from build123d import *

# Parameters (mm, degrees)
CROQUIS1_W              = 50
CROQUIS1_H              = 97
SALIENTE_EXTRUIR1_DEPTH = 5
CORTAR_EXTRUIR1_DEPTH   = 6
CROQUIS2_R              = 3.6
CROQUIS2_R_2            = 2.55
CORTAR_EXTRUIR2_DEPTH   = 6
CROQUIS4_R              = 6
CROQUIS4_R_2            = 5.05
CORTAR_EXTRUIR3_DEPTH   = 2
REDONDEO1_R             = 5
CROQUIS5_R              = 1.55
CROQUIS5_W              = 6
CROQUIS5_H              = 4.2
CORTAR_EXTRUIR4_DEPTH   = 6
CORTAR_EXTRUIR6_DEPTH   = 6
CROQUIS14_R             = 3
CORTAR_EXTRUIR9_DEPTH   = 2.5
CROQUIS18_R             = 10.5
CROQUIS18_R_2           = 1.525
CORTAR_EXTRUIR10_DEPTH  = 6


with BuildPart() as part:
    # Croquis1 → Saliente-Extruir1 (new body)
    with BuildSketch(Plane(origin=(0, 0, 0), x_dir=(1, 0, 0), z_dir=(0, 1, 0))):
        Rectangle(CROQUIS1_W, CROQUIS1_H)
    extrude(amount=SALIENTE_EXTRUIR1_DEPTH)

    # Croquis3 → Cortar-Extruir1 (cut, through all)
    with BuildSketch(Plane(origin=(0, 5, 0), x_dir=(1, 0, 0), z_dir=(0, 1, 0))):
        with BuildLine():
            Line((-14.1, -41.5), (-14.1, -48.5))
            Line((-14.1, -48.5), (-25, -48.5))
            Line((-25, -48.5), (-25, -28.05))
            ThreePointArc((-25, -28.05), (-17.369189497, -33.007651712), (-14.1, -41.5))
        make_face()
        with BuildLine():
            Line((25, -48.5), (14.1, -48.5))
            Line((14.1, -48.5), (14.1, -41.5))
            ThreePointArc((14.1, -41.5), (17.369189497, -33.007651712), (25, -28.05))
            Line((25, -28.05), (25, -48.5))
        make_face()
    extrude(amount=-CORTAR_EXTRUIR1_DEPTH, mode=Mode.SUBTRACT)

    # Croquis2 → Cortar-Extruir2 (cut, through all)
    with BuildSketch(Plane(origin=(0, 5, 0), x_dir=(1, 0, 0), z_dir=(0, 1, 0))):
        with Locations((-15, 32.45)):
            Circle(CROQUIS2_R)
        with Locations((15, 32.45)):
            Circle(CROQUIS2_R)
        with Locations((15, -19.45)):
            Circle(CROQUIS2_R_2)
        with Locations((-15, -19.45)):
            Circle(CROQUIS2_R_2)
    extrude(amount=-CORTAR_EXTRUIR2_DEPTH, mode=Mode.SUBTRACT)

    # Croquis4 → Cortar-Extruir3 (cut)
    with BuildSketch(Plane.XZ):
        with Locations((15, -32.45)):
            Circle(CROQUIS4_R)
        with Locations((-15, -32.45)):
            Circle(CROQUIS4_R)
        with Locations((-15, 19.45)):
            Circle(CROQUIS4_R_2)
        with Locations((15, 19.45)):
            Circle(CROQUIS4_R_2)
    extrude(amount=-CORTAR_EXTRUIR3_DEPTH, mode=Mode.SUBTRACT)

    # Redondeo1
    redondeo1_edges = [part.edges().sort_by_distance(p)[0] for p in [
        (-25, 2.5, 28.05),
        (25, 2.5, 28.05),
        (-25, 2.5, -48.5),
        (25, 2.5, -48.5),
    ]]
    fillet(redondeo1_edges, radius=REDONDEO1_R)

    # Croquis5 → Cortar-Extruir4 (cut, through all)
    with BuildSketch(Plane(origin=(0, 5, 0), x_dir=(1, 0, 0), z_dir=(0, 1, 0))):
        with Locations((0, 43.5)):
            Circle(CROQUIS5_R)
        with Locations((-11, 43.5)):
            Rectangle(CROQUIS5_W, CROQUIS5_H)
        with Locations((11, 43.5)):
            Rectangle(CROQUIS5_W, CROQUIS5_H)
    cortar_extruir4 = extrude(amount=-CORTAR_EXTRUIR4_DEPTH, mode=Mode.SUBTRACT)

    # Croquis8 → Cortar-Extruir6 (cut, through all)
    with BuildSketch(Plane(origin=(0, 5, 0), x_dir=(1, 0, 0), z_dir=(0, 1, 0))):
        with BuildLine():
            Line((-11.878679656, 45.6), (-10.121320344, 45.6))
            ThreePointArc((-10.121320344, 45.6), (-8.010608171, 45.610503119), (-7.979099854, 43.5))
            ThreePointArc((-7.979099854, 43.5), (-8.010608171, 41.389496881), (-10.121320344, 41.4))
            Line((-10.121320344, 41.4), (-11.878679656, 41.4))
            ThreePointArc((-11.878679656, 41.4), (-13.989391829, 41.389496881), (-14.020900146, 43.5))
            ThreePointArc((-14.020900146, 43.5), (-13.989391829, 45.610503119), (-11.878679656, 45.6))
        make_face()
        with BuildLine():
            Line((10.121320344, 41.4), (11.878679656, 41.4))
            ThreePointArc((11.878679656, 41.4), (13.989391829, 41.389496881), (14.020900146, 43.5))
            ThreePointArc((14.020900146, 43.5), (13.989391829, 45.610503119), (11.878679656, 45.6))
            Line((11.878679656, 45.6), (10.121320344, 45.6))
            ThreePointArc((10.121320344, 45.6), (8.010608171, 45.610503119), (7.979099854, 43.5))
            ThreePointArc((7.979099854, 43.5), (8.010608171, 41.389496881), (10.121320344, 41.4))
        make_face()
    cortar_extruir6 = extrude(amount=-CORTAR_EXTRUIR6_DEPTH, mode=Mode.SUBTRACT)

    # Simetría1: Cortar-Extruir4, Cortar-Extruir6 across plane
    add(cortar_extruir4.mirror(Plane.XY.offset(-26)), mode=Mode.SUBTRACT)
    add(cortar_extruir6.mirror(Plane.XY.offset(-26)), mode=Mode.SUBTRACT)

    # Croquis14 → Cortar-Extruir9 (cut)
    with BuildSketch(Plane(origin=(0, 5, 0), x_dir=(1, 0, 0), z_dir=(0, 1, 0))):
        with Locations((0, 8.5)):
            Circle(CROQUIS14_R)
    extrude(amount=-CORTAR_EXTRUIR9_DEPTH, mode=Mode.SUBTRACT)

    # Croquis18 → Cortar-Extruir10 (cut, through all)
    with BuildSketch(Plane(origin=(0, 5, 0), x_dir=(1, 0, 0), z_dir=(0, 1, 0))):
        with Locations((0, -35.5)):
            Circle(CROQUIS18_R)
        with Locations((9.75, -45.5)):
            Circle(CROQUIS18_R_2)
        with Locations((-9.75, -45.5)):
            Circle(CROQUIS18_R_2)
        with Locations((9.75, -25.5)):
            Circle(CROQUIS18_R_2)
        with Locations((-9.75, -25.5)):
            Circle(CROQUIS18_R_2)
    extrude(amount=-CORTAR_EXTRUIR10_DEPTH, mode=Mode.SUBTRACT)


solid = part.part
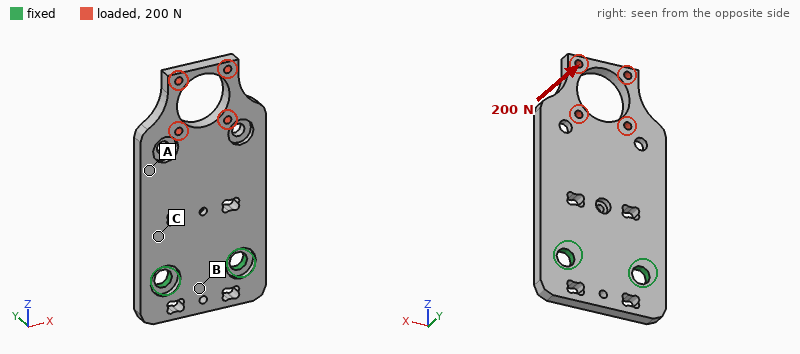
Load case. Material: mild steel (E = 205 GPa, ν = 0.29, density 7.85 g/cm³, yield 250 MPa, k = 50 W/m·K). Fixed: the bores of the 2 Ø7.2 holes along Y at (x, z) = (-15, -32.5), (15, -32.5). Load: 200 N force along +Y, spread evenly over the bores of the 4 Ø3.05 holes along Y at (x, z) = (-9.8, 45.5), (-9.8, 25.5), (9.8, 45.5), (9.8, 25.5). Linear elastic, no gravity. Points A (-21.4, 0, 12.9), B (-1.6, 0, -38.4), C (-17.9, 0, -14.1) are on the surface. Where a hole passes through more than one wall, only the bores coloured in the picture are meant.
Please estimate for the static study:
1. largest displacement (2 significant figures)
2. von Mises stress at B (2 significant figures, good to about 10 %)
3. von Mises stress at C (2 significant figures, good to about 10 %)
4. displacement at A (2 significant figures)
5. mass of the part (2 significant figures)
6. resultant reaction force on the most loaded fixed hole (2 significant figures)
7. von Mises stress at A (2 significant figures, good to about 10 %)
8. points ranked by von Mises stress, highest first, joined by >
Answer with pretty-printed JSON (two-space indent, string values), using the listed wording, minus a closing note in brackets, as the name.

{
  "largest displacement": "0.33 mm",
  "von Mises stress at B": "12 MPa",
  "von Mises stress at C": "52 MPa",
  "displacement at A": "0.13 mm",
  "mass of the part": "150 g",
  "resultant reaction force on the most loaded fixed hole": "130 N",
  "von Mises stress at A": "26 MPa",
  "points ranked by von Mises stress, highest first, joined by >": "C > A > B"
}
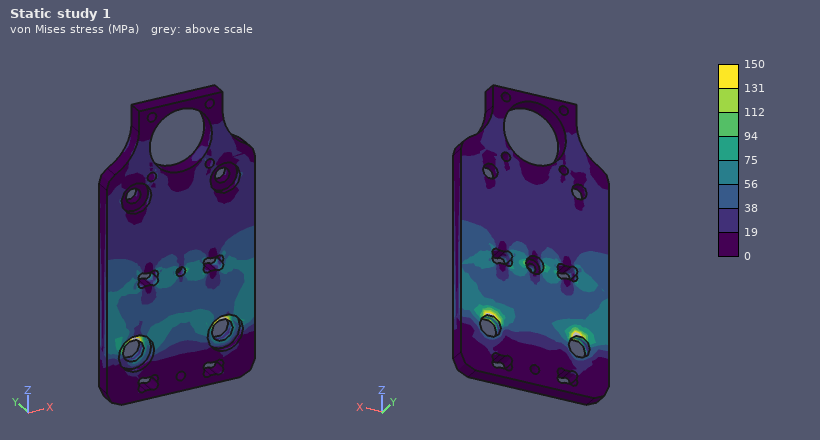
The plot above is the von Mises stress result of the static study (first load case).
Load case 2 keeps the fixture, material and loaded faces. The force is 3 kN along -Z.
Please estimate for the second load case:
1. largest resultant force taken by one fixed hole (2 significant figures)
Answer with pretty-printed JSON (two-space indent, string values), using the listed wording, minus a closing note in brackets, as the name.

{
  "largest resultant force taken by one fixed hole": "1.5 kN"
}
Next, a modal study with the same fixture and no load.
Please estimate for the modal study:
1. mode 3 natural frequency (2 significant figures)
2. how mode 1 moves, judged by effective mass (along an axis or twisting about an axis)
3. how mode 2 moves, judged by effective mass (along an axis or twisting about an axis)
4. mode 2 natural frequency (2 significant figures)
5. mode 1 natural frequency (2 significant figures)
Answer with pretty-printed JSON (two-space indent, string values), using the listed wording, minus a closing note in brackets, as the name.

{
  "mode 3 natural frequency": "3900 Hz",
  "how mode 1 moves, judged by effective mass": "along Y",
  "how mode 2 moves, judged by effective mass": "twisting about Z",
  "mode 2 natural frequency": "2700 Hz",
  "mode 1 natural frequency": "800 Hz"
}
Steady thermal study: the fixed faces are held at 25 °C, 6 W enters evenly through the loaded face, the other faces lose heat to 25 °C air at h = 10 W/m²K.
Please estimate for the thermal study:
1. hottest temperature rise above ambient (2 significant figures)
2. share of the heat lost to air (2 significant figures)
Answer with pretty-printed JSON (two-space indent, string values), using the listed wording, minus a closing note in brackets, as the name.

{
  "hottest temperature rise above ambient": "47 K",
  "share of the heat lost to air": "24 %"
}
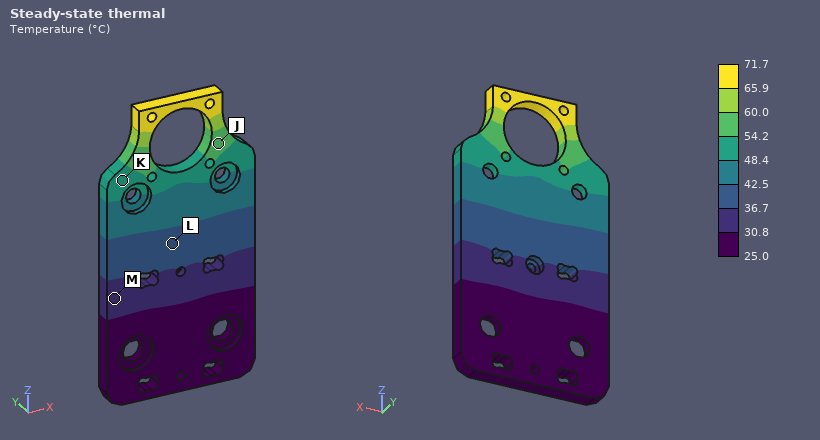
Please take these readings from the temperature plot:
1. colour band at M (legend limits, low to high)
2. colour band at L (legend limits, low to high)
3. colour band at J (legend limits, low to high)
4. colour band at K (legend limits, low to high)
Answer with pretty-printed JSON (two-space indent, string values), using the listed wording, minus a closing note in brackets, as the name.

{
  "colour band at M": "30.8 to 36.7 °C",
  "colour band at L": "36.7 to 42.5 °C",
  "colour band at J": "54.2 to 60.0 °C",
  "colour band at K": "48.4 to 54.2 °C"
}
